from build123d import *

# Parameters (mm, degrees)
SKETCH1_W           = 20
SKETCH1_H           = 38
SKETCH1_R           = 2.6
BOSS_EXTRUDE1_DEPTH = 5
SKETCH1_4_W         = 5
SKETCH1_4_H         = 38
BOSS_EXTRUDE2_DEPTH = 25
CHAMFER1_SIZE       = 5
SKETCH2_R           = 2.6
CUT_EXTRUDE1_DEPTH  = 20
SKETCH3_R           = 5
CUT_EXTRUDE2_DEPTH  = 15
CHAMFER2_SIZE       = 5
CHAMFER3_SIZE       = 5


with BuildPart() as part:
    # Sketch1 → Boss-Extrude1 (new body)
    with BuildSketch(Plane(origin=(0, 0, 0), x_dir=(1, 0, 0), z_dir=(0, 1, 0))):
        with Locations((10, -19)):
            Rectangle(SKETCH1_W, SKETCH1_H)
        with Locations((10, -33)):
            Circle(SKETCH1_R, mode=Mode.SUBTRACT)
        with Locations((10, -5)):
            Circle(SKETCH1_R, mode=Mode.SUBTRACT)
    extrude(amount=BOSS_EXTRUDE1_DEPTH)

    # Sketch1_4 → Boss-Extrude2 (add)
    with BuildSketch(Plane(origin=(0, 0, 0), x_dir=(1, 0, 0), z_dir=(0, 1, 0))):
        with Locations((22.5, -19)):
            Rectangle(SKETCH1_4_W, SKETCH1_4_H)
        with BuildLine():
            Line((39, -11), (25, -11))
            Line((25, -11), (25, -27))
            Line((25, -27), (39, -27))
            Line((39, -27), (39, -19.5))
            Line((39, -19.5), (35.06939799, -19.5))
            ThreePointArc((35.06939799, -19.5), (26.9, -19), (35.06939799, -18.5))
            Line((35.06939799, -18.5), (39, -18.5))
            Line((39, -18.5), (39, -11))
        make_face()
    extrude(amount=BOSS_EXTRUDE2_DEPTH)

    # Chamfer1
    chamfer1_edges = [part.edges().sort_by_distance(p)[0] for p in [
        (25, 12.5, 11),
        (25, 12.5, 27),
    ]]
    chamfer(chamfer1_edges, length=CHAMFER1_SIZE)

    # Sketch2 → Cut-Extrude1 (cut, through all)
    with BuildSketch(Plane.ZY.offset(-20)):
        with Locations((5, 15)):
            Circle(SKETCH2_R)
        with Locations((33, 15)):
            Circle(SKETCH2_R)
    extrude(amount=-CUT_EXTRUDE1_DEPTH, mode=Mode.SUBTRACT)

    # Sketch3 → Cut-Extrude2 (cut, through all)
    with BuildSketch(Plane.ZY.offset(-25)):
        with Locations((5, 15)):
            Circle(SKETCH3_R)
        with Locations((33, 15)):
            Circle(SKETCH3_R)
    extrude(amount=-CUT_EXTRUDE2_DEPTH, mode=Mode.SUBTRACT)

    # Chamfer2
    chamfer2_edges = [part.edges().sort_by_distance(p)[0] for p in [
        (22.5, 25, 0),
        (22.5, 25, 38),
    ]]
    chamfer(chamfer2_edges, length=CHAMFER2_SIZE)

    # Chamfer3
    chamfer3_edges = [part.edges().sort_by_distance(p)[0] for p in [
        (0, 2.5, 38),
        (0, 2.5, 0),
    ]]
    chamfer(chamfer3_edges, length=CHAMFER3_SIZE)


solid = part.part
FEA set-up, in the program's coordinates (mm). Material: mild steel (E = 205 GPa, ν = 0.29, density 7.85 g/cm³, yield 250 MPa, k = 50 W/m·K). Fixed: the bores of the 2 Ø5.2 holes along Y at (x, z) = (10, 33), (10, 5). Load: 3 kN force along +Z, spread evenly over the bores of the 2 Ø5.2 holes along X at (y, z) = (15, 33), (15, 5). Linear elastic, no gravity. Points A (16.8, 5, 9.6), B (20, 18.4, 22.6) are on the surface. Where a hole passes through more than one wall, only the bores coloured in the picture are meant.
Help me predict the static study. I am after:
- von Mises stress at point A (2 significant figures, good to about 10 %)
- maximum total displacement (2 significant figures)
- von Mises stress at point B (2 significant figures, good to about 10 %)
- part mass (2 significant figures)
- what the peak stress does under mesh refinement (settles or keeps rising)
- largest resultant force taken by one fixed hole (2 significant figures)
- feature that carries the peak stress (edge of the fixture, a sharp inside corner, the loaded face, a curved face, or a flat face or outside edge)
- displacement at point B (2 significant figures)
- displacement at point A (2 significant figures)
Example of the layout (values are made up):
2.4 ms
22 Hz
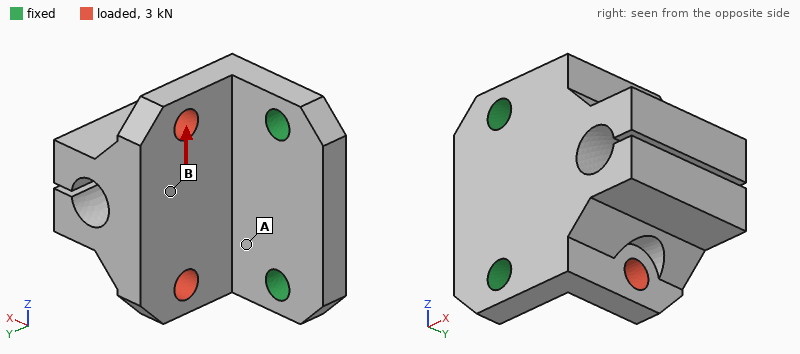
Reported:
87 MPa
27 µm
24 MPa
99 g
keeps rising
2.3 kN
edge of the fixture
19 µm
4.1 µm
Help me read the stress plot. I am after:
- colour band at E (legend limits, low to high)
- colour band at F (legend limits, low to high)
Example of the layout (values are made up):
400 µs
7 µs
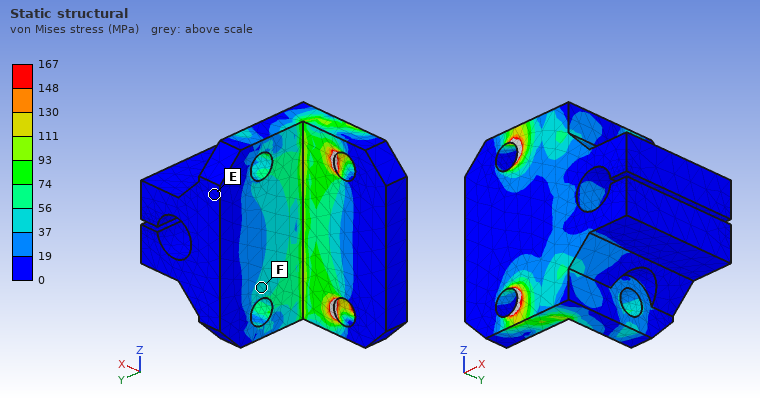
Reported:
0 to 19 MPa
37 to 56 MPa
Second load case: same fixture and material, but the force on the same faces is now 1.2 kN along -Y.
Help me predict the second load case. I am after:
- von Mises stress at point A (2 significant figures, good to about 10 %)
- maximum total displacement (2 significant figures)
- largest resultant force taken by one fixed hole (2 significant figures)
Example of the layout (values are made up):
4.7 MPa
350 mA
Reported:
39 MPa
37 µm
600 N
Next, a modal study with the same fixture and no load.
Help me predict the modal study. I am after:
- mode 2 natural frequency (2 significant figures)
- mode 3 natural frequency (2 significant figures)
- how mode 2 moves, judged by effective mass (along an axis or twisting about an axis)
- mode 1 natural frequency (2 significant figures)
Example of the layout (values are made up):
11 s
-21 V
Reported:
8300 Hz
12 kHz
along Z
2700 Hz
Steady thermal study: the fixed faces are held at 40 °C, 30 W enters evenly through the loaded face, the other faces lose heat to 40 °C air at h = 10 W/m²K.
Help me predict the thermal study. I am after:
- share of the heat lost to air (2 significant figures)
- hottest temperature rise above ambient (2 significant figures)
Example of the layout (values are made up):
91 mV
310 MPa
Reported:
7.4 %
78 K
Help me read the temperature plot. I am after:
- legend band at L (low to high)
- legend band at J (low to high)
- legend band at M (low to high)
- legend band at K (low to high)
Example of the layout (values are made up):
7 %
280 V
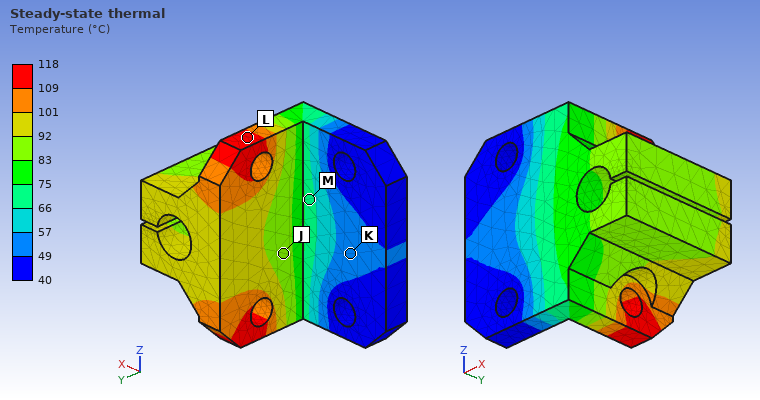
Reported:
109 to 118 °C
83 to 92 °C
66 to 75 °C
49 to 57 °C
